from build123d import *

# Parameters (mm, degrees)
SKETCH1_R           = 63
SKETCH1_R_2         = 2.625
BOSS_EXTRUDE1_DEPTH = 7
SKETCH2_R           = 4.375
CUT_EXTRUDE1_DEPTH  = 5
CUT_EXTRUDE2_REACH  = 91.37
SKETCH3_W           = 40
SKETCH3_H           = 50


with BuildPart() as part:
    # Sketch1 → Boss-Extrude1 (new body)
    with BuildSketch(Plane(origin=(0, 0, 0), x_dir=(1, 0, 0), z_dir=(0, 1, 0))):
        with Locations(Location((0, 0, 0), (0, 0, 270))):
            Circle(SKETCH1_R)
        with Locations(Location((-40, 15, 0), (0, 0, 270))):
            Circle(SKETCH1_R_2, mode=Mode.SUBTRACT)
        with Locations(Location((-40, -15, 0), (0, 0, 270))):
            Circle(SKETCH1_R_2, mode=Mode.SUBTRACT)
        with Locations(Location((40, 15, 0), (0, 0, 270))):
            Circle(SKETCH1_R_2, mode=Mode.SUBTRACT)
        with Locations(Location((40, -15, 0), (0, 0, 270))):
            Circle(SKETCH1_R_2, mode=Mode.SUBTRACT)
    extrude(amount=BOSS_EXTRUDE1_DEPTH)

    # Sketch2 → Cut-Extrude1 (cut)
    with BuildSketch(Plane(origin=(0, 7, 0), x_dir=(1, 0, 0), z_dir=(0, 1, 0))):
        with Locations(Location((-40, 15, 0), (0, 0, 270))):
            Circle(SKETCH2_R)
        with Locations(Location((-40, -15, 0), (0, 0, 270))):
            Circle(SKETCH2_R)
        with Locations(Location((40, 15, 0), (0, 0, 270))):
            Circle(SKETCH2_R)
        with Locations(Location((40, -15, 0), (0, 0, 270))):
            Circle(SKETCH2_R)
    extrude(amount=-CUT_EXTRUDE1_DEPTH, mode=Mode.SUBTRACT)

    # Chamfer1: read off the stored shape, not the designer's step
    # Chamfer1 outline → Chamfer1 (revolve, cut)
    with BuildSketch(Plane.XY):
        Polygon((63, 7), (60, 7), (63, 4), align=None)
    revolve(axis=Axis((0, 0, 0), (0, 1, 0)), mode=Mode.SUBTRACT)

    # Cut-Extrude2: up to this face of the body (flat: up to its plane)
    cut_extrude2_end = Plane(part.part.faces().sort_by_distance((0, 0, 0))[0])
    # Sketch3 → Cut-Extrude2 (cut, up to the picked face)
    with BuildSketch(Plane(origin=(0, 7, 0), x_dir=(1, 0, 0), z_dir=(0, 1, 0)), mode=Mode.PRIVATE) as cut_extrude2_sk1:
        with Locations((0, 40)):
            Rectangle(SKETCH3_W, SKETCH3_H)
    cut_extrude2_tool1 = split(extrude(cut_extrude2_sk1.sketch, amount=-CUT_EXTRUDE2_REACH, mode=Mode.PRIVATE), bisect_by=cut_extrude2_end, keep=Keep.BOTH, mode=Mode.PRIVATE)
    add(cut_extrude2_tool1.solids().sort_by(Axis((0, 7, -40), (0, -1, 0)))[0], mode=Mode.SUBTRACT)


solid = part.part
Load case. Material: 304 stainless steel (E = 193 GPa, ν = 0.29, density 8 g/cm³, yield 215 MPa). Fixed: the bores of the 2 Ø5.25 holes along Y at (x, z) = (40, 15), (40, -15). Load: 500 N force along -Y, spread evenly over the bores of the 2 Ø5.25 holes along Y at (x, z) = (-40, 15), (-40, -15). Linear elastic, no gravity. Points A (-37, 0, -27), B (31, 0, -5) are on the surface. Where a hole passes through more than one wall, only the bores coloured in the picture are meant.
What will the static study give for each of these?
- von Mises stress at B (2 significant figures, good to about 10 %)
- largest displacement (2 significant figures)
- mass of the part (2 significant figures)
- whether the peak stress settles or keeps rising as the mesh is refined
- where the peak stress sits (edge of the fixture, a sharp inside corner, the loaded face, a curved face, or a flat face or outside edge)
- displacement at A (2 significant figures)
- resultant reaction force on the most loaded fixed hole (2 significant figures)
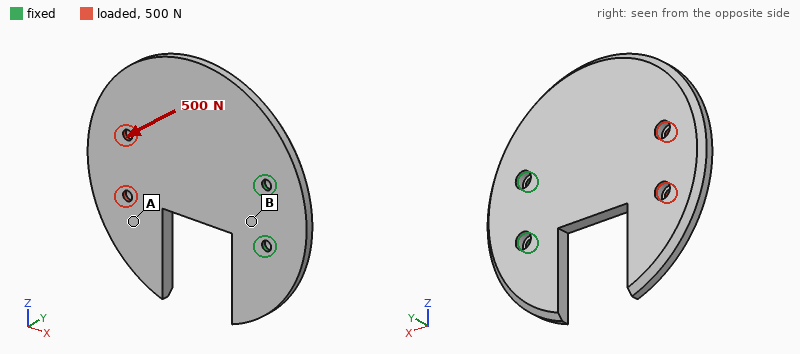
68 MPa
0.74 mm
570 g
keeps rising
edge of the fixture
0.53 mm
450 N
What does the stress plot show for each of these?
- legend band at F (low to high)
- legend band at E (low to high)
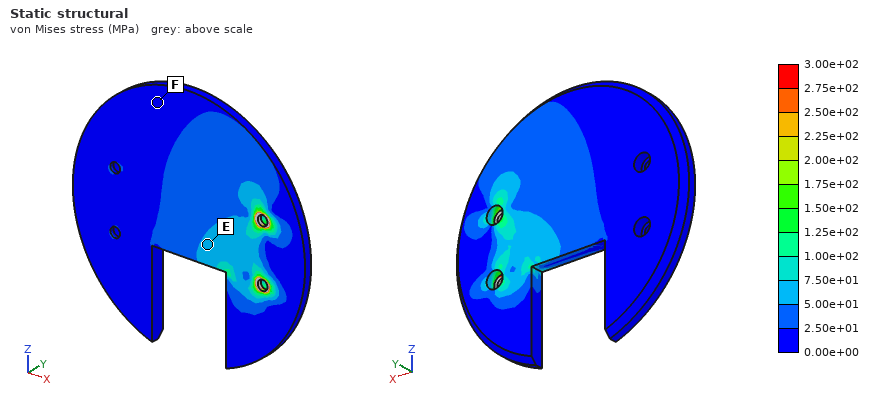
0.00e+00 to 2.50e+01 MPa
5.00e+01 to 7.50e+01 MPa
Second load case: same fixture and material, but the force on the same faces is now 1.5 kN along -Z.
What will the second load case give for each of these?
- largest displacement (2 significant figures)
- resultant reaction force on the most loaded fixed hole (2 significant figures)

65 µm
3.8 kN
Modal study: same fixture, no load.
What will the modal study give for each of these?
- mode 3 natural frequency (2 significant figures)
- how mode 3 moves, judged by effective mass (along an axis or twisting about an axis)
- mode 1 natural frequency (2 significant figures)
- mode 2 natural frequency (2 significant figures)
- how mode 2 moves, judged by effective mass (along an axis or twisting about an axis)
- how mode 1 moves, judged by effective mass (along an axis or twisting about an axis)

1900 Hz
along Z
320 Hz
900 Hz
twisting about X
along Y
